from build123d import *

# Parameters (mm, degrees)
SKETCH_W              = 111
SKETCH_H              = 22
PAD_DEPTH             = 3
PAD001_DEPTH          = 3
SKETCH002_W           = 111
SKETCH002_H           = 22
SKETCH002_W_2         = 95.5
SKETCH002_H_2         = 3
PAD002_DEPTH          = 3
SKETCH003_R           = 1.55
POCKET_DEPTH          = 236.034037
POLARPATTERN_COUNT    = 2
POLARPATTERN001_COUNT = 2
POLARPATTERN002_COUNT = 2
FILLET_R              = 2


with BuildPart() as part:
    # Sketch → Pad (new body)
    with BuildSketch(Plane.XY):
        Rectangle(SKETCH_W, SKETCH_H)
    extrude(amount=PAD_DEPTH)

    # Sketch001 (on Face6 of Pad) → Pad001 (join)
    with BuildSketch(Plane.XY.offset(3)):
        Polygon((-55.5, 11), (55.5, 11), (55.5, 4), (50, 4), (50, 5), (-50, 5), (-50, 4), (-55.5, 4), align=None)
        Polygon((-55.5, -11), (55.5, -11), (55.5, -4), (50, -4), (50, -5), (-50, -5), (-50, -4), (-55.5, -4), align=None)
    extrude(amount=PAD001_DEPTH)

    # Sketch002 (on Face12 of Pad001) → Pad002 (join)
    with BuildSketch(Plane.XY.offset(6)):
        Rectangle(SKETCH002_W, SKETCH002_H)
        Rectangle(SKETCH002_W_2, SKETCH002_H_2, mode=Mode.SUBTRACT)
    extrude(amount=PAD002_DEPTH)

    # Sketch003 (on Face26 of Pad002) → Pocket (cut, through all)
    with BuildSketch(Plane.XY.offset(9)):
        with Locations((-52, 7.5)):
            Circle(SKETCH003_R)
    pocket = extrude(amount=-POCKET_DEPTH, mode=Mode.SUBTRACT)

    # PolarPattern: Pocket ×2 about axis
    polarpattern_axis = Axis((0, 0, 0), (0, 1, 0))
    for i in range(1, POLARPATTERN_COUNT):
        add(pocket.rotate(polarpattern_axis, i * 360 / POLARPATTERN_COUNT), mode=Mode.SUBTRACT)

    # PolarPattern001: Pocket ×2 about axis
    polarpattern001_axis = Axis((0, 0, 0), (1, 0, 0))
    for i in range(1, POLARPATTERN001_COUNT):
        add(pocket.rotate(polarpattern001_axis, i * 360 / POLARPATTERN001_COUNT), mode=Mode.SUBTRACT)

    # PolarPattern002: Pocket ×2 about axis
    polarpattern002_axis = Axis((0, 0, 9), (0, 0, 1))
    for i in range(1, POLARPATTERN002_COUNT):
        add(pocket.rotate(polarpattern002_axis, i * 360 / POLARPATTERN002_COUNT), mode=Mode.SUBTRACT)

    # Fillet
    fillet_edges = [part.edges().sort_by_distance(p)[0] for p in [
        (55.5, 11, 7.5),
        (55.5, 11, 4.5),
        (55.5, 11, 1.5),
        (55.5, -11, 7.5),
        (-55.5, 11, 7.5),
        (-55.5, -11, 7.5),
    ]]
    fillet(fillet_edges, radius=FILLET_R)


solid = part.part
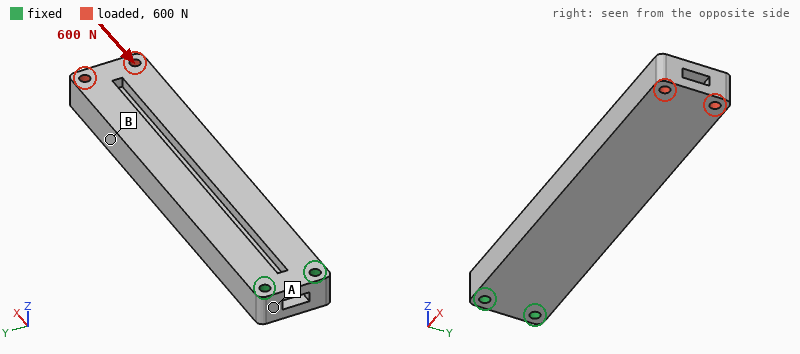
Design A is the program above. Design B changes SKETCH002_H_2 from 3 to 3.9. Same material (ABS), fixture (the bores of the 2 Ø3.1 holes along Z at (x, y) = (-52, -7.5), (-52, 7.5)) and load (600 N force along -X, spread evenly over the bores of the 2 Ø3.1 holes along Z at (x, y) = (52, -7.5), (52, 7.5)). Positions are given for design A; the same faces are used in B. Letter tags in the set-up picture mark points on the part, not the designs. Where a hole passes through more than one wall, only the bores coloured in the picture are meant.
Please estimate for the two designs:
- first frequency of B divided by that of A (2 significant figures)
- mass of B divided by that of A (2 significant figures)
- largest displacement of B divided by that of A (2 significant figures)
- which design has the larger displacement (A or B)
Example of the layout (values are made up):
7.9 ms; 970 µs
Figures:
1.00; 0.99; 1.2; B
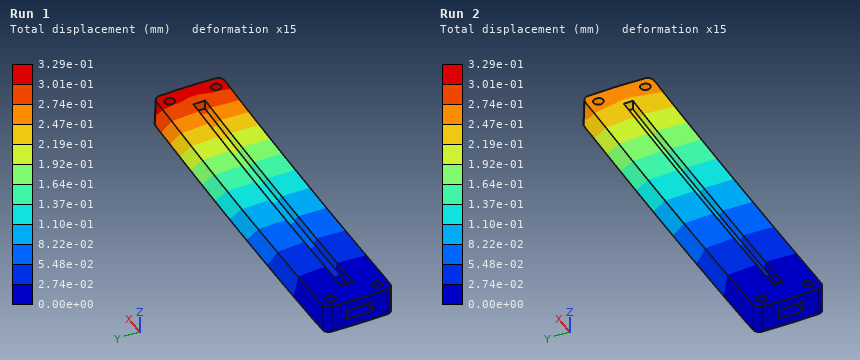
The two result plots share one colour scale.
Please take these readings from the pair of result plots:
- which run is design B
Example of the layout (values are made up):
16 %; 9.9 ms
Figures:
Run 1
